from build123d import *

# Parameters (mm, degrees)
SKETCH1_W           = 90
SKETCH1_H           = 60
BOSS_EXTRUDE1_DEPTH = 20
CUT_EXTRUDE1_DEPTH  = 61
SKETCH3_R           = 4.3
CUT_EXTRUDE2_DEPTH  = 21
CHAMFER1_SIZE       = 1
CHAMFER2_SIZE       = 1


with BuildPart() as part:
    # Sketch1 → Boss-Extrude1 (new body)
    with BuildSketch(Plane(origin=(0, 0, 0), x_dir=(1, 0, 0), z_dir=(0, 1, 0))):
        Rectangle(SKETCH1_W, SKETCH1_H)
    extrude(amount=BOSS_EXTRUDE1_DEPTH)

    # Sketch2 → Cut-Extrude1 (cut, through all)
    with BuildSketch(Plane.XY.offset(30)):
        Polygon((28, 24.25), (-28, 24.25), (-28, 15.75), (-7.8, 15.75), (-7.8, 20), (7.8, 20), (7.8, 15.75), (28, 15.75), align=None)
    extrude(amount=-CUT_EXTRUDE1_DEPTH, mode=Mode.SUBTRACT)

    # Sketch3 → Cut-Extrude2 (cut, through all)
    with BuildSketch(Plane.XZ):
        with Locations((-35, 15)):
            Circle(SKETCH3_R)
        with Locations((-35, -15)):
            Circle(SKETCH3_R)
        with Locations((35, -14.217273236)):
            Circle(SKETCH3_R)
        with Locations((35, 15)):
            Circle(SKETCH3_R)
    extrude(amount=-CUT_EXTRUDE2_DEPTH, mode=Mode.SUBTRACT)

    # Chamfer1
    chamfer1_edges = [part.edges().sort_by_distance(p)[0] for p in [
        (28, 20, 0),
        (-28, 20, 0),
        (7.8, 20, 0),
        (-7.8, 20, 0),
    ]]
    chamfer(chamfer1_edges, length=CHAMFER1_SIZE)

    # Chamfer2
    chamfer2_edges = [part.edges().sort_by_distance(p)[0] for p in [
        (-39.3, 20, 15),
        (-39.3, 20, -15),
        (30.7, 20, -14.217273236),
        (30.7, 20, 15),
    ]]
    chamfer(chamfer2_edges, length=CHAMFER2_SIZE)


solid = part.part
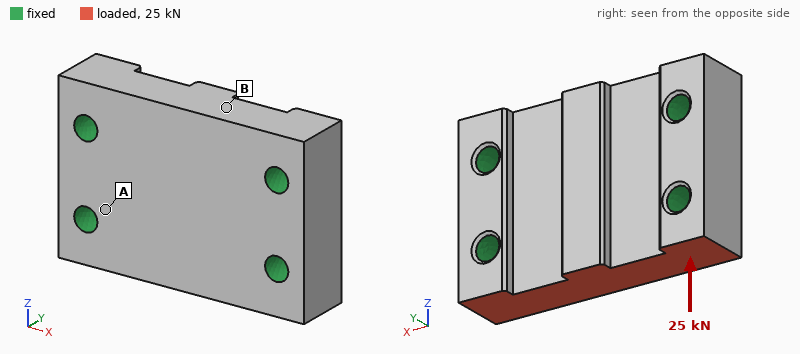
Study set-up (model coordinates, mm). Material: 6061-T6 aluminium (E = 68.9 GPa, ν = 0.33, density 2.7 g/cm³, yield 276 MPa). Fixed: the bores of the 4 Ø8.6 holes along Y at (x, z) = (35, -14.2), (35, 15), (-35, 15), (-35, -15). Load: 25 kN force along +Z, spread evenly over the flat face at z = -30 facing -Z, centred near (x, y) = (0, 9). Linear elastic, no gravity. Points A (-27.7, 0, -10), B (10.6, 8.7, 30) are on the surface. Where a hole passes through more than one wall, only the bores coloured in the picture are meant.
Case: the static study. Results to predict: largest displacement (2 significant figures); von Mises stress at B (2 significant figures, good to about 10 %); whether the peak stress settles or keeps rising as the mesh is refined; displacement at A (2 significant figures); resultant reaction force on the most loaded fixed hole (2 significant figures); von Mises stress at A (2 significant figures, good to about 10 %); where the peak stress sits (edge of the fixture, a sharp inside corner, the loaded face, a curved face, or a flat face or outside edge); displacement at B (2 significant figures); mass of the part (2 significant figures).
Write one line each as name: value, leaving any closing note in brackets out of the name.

largest displacement: 14 µm
von Mises stress at B: 8.0 MPa
whether the peak stress settles or keeps rising as the mesh is refined: keeps rising
displacement at A: 2.3 µm
resultant reaction force on the most loaded fixed hole: 9.3 kN
von Mises stress at A: 18 MPa
where the peak stress sits: edge of the fixture
displacement at B: 5.5 µm
mass of the part: 250 g
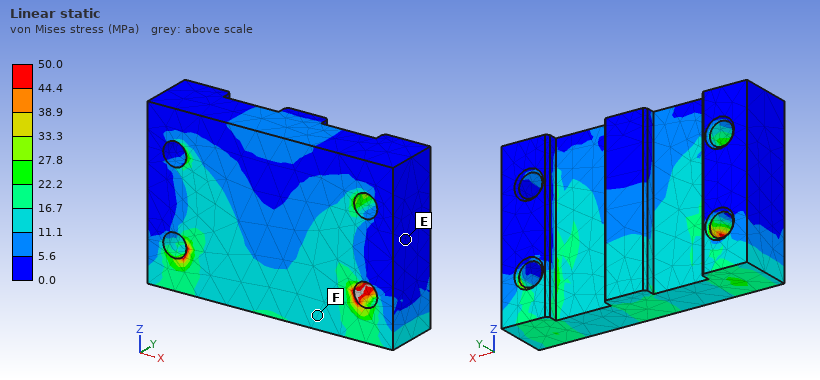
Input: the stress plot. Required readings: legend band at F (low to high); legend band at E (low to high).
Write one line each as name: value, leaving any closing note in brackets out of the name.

legend band at F: 11.1 to 16.7 MPa
legend band at E: 0.0 to 5.6 MPa
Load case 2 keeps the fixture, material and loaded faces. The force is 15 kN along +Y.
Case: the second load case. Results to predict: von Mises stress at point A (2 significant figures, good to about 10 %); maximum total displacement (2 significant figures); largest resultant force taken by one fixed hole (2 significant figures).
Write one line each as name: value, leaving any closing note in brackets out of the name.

von Mises stress at point A: 29 MPa
maximum total displacement: 47 µm
largest resultant force taken by one fixed hole: 8.3 kN
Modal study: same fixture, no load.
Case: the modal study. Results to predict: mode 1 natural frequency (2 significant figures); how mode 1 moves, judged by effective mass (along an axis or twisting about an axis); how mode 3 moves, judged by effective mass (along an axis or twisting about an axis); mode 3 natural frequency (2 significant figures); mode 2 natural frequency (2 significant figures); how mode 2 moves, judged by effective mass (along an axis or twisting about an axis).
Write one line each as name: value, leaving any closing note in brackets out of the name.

mode 1 natural frequency: 14 kHz
how mode 1 moves, judged by effective mass: along Y
how mode 3 moves, judged by effective mass: along Z
mode 3 natural frequency: 19 kHz
mode 2 natural frequency: 15 kHz
how mode 2 moves, judged by effective mass: twisting about X
